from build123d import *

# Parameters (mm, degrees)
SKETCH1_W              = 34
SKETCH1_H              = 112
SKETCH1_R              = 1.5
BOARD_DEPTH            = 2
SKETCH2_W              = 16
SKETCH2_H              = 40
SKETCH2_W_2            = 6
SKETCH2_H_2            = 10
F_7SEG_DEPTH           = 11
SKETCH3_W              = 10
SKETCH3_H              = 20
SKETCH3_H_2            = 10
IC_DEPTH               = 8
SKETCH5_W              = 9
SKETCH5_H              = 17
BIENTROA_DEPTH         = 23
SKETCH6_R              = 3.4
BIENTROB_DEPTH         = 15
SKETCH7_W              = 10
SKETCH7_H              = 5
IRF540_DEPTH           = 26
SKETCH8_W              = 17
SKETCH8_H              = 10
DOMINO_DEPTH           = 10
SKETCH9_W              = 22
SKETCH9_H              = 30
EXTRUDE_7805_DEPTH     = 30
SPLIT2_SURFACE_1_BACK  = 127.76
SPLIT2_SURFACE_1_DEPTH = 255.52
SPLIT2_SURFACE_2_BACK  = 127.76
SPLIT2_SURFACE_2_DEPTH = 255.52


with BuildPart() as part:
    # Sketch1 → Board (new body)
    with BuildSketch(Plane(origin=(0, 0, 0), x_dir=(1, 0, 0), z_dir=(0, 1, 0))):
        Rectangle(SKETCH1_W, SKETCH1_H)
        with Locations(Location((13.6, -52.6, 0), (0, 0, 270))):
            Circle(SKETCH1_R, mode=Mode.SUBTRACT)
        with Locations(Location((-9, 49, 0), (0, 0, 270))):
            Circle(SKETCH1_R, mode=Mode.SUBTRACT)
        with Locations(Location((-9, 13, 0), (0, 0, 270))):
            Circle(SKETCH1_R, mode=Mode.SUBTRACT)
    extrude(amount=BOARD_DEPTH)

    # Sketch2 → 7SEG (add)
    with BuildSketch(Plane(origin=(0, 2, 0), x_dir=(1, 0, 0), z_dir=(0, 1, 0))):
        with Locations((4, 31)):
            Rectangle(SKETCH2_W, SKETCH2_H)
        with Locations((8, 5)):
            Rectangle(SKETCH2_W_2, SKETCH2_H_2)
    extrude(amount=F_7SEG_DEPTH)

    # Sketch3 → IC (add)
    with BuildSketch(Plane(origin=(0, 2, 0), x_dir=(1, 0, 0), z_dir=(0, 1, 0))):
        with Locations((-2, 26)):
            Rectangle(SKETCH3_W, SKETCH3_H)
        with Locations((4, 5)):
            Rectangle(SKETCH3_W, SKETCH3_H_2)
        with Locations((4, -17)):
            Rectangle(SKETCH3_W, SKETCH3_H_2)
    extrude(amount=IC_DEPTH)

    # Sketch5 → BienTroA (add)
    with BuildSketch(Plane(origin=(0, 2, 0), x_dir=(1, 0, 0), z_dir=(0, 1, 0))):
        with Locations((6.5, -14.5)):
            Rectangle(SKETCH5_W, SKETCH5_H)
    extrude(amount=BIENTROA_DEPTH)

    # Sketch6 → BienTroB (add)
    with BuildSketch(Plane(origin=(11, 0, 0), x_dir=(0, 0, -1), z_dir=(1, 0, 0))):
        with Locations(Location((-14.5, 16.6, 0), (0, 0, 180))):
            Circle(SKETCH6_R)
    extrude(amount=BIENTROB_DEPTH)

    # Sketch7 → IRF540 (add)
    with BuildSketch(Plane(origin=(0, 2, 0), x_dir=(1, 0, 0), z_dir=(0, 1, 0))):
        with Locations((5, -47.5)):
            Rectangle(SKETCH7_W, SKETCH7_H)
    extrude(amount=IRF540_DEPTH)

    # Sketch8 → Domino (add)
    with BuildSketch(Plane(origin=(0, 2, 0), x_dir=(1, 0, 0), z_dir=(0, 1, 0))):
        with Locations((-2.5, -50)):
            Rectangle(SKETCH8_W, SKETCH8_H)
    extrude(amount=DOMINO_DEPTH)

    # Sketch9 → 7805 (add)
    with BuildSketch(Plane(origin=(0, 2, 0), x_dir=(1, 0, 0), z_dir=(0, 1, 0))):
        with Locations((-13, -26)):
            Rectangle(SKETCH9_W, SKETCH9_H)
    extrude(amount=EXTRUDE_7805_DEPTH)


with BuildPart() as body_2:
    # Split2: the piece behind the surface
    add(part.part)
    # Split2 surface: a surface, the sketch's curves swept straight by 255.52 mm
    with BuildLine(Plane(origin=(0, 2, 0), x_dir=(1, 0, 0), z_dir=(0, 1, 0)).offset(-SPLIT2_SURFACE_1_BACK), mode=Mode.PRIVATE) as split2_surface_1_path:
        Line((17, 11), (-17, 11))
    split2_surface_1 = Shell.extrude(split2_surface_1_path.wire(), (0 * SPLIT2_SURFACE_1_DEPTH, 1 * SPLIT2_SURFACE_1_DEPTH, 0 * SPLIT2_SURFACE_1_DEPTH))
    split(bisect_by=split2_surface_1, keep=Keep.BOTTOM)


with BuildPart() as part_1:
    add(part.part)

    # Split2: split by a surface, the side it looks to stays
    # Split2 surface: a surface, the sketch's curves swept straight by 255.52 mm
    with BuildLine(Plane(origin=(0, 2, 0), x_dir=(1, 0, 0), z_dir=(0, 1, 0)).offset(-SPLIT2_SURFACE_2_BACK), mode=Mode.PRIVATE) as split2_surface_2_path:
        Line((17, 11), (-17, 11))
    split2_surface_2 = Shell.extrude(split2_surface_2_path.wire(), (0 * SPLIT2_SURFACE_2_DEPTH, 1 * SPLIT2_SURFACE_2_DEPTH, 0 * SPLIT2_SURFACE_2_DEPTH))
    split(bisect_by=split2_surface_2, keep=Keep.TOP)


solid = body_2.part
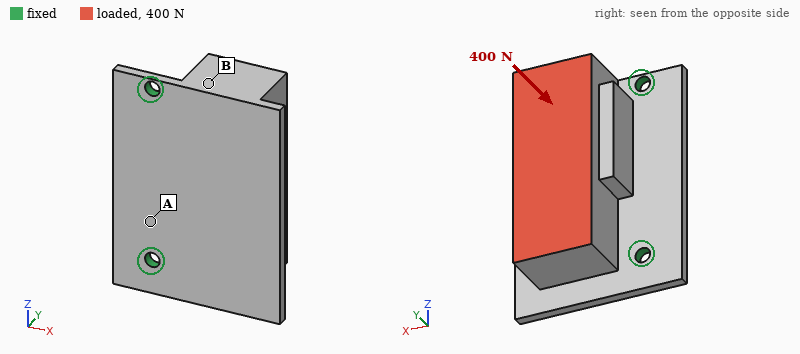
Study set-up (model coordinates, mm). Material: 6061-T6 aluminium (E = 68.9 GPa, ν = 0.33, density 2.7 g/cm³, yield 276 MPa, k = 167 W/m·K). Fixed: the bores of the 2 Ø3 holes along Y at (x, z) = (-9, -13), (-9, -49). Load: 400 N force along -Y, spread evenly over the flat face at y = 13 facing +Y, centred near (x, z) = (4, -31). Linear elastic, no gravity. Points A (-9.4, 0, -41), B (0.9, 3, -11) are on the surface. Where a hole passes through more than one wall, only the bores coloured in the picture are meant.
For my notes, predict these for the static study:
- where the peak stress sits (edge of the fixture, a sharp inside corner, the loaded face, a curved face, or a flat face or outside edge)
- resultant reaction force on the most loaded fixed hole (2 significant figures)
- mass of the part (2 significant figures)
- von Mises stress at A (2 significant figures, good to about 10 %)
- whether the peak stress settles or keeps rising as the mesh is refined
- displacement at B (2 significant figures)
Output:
edge of the fixture
210 N
28 g
61 MPa
keeps rising
0.11 mm
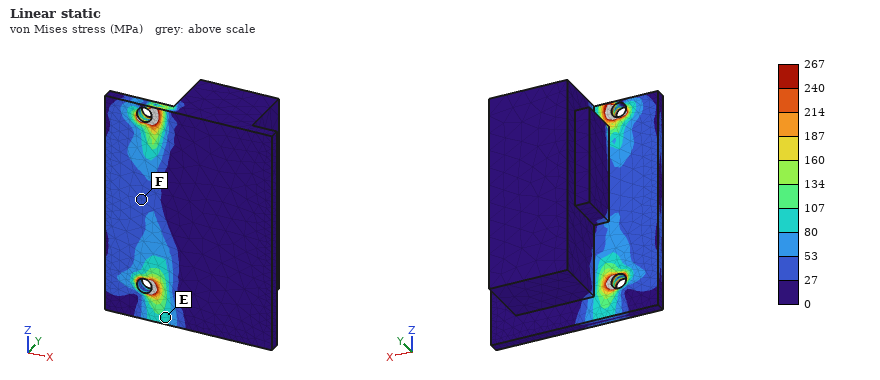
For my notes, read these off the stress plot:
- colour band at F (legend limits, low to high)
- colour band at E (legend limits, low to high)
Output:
27 to 53 MPa
80 to 107 MPa
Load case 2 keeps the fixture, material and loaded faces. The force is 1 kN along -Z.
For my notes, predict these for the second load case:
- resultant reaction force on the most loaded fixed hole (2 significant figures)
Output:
710 N
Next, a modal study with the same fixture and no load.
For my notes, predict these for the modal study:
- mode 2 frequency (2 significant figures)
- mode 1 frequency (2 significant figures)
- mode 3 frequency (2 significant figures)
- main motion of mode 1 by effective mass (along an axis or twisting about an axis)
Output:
8300 Hz
1300 Hz
11 kHz
along Y
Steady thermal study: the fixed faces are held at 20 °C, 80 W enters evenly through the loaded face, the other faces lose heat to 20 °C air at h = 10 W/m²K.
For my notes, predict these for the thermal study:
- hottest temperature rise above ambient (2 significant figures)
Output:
72 K
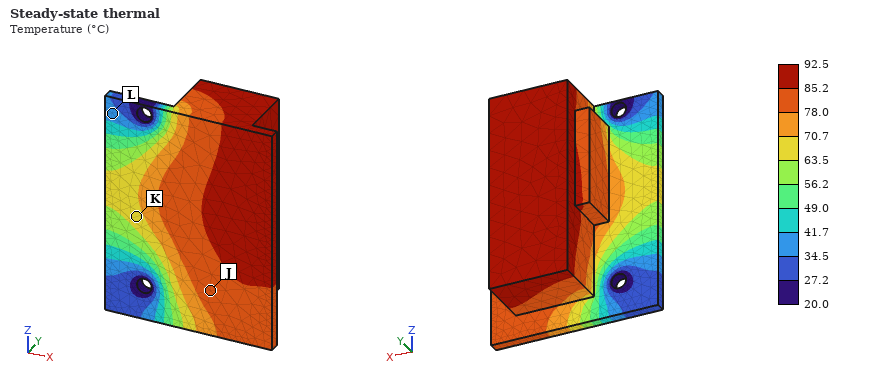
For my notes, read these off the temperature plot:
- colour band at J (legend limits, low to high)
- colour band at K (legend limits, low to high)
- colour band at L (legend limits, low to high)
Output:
78.0 to 85.2 °C
63.5 to 70.7 °C
34.5 to 41.7 °C
